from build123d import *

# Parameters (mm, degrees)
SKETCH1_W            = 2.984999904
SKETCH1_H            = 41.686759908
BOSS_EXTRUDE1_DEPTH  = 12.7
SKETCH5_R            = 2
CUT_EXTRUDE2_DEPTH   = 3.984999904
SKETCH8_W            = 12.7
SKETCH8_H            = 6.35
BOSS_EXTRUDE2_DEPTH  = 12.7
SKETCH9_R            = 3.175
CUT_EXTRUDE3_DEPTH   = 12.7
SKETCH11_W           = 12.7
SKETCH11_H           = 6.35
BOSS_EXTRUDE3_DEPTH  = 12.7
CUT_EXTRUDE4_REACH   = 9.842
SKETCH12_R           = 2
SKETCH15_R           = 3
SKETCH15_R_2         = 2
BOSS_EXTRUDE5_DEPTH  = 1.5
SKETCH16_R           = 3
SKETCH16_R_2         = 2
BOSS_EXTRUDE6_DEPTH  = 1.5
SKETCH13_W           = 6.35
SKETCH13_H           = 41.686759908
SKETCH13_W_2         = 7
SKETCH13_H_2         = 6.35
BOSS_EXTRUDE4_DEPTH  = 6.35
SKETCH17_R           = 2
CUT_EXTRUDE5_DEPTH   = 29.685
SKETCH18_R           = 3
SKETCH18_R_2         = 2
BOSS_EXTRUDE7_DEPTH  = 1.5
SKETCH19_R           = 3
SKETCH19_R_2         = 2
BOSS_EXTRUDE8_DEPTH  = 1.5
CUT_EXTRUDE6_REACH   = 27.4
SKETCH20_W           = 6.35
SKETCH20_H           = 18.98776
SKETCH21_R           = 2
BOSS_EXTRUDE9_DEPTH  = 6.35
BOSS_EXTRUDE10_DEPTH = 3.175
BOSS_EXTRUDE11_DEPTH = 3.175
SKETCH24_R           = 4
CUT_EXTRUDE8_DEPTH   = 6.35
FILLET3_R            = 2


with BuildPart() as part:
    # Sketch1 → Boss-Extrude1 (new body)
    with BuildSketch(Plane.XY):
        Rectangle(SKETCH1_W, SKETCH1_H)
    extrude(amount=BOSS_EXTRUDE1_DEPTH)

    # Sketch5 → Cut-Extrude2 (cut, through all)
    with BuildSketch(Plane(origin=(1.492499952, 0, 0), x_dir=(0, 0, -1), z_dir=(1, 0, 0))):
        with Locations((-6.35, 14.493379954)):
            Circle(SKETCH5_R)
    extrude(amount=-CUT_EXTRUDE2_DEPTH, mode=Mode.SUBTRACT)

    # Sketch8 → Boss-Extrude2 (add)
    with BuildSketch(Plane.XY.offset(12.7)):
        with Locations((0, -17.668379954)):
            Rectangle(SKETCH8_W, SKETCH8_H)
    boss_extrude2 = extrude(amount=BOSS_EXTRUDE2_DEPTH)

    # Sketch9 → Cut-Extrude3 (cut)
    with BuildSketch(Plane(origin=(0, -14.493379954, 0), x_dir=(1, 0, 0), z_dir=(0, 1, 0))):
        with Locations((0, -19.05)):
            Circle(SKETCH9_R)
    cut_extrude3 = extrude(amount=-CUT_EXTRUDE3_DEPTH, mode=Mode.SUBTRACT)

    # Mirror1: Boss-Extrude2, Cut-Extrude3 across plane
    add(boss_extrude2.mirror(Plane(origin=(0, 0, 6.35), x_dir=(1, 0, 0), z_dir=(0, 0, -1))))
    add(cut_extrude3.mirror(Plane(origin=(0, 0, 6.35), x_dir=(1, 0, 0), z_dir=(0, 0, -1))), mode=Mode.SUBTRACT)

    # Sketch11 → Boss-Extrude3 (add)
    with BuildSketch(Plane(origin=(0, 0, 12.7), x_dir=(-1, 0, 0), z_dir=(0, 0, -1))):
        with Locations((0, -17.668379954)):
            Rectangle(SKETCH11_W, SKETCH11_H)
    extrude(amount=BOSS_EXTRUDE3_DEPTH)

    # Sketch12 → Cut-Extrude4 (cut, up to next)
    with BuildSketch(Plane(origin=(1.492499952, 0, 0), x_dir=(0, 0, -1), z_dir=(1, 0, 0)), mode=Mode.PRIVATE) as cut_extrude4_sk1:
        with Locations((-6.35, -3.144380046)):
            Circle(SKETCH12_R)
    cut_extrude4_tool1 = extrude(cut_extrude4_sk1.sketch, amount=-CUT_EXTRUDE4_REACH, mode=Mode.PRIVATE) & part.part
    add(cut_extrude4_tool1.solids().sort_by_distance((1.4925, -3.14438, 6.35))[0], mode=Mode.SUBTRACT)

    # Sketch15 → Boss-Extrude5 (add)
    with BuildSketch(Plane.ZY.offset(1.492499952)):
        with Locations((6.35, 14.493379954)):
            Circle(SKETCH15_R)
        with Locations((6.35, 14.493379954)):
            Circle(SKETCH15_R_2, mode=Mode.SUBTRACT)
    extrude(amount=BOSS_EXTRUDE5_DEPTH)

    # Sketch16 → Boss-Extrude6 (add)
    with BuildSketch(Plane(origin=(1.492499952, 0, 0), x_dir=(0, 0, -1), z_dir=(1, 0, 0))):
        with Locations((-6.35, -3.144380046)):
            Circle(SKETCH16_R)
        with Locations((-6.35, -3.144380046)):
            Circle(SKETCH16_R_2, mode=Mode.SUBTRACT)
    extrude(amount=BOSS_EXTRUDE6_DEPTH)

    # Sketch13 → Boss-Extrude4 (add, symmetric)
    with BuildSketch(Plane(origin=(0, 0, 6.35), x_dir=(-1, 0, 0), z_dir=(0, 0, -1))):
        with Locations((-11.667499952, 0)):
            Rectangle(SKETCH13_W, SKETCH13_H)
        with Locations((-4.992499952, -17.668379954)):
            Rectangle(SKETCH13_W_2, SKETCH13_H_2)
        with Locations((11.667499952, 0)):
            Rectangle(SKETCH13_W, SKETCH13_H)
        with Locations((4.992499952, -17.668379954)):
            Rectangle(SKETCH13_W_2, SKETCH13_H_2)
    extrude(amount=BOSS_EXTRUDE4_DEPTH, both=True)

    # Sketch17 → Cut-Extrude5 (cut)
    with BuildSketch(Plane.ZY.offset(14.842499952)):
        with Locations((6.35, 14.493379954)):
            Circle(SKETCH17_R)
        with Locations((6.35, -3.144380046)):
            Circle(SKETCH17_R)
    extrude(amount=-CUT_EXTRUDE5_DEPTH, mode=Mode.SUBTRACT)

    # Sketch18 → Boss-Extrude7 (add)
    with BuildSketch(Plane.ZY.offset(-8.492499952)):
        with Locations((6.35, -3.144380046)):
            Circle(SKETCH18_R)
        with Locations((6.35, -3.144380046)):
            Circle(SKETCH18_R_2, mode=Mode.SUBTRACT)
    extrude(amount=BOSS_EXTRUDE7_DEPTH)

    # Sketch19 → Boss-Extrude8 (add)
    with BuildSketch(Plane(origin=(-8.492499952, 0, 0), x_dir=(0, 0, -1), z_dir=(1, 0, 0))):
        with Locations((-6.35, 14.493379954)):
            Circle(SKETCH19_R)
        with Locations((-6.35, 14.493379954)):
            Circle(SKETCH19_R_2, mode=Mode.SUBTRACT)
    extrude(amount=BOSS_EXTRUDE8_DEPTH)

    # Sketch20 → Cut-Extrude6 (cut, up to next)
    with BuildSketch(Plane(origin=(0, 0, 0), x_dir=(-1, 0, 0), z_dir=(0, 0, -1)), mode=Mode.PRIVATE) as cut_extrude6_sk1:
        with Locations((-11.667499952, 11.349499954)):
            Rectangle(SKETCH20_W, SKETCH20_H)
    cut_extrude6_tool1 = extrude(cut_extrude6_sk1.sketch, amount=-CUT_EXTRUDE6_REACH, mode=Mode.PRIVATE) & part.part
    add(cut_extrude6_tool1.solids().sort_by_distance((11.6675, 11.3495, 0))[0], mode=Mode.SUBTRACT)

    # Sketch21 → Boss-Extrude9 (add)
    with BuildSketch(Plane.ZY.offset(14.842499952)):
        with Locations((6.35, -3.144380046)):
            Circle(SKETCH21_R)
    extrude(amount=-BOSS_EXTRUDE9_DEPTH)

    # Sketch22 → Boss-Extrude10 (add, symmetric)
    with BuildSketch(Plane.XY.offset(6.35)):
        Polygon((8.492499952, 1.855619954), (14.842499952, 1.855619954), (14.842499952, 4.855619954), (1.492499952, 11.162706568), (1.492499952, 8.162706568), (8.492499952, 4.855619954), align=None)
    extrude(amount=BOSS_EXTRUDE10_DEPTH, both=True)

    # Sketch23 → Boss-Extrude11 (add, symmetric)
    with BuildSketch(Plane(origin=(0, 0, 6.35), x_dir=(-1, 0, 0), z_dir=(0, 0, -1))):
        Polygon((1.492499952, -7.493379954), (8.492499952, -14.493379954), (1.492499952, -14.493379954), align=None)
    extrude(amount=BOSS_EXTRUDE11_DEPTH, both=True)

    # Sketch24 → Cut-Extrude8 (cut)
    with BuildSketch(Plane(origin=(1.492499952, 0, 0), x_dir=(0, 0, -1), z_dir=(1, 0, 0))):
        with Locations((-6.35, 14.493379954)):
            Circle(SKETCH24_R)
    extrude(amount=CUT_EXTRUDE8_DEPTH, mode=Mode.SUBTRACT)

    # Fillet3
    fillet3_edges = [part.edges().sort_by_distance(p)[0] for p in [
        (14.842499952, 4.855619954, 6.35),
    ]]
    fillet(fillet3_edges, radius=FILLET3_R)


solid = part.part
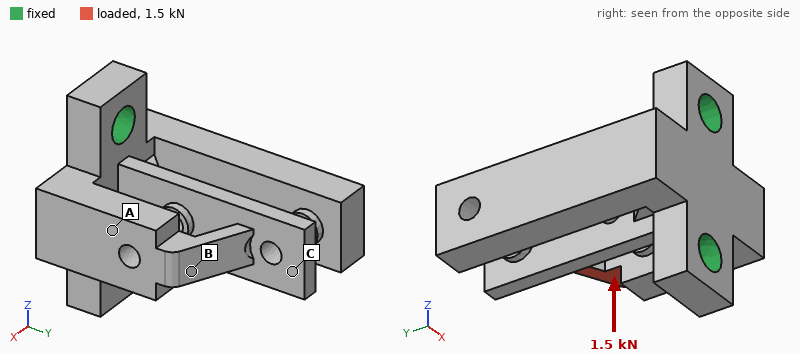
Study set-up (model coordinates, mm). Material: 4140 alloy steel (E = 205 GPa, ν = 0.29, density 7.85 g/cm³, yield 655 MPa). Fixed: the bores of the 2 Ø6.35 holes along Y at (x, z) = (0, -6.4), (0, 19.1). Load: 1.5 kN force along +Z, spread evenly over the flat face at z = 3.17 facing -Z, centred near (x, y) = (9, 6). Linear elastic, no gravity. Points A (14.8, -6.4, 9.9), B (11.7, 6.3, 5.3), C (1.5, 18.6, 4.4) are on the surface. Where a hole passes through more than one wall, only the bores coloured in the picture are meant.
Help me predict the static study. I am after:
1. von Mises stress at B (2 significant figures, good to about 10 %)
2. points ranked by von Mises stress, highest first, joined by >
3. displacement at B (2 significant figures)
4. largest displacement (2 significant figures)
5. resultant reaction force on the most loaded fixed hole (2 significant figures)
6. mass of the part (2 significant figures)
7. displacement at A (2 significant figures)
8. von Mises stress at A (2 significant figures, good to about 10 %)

61 MPa
B > A > C
58 µm
73 µm
2.2 kN
78 g
26 µm
35 MPa
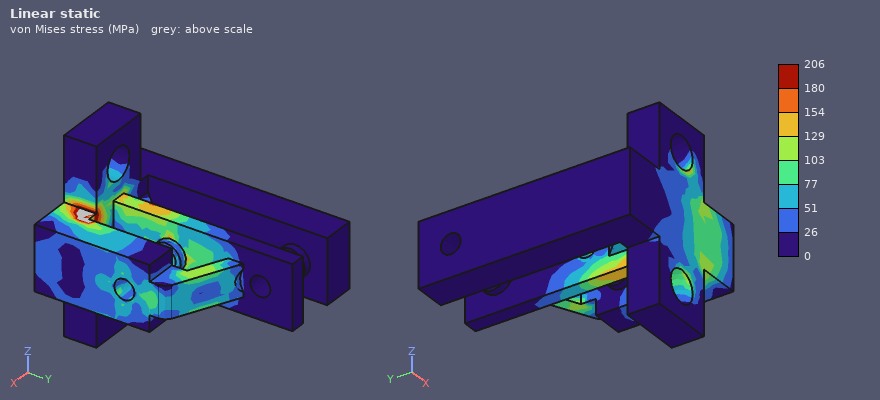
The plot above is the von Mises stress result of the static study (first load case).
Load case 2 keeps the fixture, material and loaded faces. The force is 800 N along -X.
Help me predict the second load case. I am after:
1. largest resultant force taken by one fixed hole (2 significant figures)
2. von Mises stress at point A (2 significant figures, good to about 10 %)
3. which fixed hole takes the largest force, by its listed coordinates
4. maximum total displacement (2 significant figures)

520 N
48 MPa
(0, -6.4)
0.11 mm
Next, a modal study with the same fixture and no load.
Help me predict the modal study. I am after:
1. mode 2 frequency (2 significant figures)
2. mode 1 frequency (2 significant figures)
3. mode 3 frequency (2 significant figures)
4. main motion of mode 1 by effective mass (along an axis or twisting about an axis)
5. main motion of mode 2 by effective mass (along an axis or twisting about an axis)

4200 Hz
2600 Hz
4500 Hz
along X
along Z
